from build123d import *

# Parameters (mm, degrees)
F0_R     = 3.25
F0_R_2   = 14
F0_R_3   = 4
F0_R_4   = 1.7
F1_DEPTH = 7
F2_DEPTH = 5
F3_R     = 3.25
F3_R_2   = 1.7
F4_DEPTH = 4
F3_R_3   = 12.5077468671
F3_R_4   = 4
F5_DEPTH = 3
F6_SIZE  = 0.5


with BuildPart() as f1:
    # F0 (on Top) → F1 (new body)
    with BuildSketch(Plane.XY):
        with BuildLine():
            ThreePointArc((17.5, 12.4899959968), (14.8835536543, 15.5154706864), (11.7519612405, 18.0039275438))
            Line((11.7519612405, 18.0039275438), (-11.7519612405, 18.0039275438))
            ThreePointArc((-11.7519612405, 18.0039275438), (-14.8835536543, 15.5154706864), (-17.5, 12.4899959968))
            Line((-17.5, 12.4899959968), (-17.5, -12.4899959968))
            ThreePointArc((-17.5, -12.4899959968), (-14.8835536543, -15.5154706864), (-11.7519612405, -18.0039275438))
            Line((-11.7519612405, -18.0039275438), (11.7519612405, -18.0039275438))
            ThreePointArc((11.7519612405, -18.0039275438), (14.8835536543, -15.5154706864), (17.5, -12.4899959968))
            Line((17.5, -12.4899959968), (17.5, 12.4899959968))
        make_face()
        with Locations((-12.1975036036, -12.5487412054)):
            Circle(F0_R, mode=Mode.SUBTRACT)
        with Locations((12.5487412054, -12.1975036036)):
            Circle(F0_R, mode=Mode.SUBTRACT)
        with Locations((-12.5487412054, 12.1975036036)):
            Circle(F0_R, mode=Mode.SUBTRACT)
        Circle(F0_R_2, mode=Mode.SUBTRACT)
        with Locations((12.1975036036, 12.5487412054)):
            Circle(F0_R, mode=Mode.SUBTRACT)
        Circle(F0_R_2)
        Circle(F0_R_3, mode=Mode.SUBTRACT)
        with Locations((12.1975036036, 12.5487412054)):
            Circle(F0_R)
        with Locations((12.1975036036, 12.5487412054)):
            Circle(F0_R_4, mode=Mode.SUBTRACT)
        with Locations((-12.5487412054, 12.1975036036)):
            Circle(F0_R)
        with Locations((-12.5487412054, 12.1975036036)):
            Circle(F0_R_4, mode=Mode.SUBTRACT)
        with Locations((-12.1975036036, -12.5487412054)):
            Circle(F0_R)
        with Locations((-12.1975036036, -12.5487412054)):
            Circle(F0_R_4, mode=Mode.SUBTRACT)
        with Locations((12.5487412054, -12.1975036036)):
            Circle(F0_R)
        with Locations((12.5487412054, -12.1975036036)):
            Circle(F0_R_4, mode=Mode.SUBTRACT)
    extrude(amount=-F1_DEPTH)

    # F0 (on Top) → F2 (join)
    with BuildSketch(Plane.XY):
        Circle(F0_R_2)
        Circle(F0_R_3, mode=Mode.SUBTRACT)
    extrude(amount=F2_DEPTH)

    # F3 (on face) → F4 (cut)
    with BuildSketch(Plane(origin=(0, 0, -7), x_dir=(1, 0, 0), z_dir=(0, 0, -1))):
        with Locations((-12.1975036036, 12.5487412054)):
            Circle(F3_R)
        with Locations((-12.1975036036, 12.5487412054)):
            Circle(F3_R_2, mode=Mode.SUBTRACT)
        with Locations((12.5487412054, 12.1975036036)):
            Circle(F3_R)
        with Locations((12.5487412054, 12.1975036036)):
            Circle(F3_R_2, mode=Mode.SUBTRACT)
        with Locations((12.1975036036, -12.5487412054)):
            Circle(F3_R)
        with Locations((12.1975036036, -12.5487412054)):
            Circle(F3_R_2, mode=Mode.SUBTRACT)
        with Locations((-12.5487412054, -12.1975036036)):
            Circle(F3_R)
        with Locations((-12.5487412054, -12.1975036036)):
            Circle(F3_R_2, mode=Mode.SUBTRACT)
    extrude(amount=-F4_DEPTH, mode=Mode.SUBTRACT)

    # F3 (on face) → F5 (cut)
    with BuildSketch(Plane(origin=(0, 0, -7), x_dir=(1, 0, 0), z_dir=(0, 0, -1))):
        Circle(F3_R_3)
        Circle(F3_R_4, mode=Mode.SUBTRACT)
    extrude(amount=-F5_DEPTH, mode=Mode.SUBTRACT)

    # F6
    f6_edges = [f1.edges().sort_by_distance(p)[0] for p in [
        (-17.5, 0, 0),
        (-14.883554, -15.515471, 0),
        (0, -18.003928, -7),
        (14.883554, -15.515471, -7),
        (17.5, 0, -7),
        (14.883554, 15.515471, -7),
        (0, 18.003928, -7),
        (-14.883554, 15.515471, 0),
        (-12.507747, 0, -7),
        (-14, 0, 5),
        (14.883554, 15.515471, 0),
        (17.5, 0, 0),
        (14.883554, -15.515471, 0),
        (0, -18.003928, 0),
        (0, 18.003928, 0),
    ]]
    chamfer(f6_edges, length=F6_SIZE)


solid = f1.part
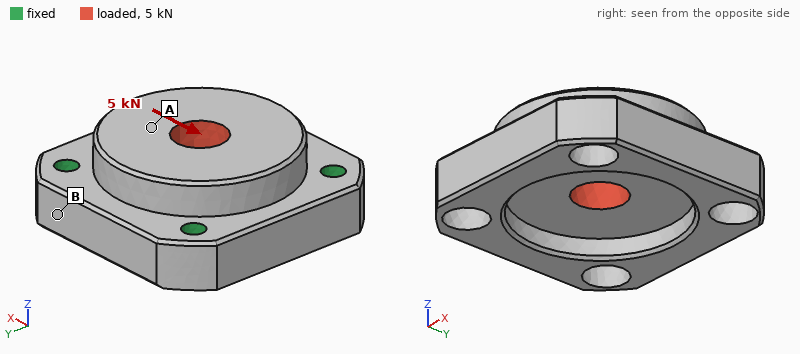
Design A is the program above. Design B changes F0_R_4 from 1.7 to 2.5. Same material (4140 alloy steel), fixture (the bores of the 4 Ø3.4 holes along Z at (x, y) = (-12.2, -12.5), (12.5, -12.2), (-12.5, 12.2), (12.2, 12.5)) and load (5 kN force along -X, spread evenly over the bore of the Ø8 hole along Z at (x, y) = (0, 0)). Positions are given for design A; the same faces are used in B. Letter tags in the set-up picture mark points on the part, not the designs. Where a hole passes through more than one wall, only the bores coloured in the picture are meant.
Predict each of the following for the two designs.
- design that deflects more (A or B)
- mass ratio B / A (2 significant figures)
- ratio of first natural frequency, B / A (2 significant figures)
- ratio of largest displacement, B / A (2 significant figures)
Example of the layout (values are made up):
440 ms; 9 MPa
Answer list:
A; 0.99; 1.2; 0.85
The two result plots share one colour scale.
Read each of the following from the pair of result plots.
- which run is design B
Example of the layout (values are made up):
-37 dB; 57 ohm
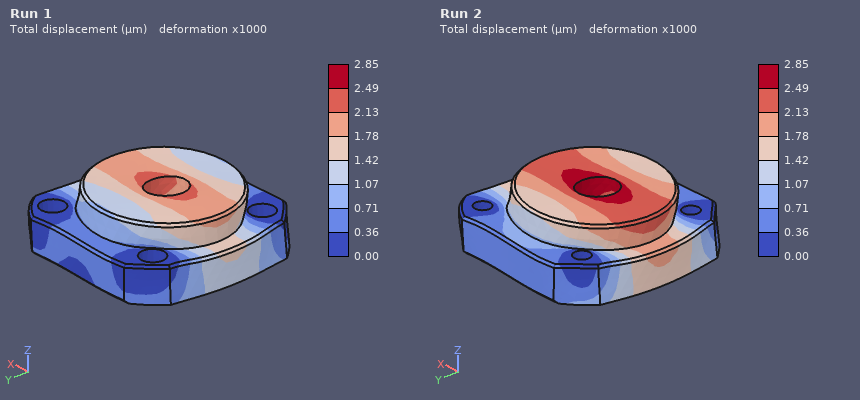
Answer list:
Run 1
